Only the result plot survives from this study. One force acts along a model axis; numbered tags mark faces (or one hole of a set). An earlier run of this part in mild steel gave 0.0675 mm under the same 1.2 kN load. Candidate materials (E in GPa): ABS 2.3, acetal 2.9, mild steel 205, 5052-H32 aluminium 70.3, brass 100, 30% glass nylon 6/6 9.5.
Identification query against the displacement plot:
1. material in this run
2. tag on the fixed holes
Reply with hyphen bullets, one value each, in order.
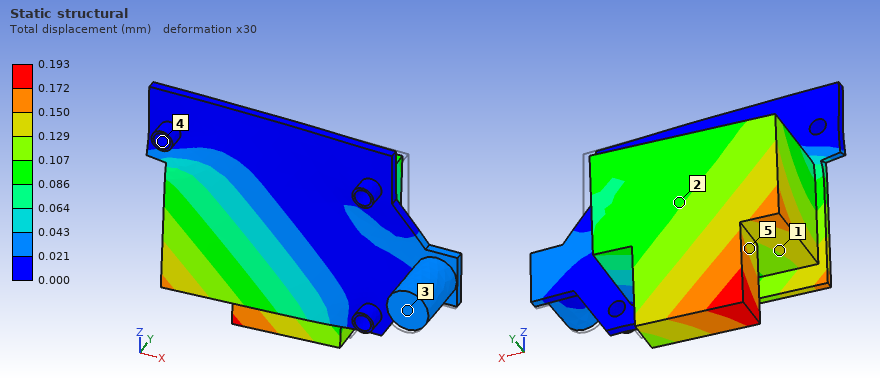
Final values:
- 5052-H32 aluminium
- 4
